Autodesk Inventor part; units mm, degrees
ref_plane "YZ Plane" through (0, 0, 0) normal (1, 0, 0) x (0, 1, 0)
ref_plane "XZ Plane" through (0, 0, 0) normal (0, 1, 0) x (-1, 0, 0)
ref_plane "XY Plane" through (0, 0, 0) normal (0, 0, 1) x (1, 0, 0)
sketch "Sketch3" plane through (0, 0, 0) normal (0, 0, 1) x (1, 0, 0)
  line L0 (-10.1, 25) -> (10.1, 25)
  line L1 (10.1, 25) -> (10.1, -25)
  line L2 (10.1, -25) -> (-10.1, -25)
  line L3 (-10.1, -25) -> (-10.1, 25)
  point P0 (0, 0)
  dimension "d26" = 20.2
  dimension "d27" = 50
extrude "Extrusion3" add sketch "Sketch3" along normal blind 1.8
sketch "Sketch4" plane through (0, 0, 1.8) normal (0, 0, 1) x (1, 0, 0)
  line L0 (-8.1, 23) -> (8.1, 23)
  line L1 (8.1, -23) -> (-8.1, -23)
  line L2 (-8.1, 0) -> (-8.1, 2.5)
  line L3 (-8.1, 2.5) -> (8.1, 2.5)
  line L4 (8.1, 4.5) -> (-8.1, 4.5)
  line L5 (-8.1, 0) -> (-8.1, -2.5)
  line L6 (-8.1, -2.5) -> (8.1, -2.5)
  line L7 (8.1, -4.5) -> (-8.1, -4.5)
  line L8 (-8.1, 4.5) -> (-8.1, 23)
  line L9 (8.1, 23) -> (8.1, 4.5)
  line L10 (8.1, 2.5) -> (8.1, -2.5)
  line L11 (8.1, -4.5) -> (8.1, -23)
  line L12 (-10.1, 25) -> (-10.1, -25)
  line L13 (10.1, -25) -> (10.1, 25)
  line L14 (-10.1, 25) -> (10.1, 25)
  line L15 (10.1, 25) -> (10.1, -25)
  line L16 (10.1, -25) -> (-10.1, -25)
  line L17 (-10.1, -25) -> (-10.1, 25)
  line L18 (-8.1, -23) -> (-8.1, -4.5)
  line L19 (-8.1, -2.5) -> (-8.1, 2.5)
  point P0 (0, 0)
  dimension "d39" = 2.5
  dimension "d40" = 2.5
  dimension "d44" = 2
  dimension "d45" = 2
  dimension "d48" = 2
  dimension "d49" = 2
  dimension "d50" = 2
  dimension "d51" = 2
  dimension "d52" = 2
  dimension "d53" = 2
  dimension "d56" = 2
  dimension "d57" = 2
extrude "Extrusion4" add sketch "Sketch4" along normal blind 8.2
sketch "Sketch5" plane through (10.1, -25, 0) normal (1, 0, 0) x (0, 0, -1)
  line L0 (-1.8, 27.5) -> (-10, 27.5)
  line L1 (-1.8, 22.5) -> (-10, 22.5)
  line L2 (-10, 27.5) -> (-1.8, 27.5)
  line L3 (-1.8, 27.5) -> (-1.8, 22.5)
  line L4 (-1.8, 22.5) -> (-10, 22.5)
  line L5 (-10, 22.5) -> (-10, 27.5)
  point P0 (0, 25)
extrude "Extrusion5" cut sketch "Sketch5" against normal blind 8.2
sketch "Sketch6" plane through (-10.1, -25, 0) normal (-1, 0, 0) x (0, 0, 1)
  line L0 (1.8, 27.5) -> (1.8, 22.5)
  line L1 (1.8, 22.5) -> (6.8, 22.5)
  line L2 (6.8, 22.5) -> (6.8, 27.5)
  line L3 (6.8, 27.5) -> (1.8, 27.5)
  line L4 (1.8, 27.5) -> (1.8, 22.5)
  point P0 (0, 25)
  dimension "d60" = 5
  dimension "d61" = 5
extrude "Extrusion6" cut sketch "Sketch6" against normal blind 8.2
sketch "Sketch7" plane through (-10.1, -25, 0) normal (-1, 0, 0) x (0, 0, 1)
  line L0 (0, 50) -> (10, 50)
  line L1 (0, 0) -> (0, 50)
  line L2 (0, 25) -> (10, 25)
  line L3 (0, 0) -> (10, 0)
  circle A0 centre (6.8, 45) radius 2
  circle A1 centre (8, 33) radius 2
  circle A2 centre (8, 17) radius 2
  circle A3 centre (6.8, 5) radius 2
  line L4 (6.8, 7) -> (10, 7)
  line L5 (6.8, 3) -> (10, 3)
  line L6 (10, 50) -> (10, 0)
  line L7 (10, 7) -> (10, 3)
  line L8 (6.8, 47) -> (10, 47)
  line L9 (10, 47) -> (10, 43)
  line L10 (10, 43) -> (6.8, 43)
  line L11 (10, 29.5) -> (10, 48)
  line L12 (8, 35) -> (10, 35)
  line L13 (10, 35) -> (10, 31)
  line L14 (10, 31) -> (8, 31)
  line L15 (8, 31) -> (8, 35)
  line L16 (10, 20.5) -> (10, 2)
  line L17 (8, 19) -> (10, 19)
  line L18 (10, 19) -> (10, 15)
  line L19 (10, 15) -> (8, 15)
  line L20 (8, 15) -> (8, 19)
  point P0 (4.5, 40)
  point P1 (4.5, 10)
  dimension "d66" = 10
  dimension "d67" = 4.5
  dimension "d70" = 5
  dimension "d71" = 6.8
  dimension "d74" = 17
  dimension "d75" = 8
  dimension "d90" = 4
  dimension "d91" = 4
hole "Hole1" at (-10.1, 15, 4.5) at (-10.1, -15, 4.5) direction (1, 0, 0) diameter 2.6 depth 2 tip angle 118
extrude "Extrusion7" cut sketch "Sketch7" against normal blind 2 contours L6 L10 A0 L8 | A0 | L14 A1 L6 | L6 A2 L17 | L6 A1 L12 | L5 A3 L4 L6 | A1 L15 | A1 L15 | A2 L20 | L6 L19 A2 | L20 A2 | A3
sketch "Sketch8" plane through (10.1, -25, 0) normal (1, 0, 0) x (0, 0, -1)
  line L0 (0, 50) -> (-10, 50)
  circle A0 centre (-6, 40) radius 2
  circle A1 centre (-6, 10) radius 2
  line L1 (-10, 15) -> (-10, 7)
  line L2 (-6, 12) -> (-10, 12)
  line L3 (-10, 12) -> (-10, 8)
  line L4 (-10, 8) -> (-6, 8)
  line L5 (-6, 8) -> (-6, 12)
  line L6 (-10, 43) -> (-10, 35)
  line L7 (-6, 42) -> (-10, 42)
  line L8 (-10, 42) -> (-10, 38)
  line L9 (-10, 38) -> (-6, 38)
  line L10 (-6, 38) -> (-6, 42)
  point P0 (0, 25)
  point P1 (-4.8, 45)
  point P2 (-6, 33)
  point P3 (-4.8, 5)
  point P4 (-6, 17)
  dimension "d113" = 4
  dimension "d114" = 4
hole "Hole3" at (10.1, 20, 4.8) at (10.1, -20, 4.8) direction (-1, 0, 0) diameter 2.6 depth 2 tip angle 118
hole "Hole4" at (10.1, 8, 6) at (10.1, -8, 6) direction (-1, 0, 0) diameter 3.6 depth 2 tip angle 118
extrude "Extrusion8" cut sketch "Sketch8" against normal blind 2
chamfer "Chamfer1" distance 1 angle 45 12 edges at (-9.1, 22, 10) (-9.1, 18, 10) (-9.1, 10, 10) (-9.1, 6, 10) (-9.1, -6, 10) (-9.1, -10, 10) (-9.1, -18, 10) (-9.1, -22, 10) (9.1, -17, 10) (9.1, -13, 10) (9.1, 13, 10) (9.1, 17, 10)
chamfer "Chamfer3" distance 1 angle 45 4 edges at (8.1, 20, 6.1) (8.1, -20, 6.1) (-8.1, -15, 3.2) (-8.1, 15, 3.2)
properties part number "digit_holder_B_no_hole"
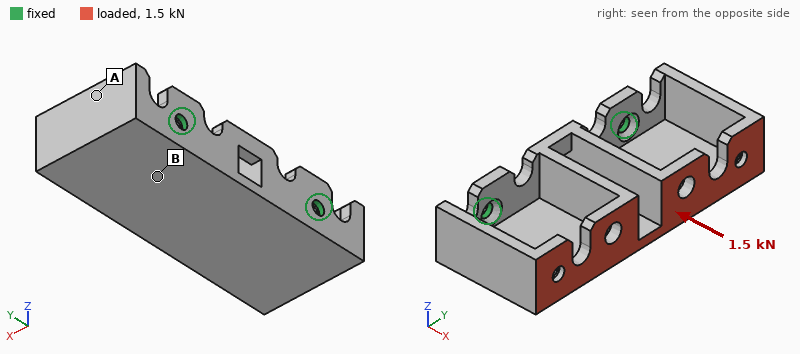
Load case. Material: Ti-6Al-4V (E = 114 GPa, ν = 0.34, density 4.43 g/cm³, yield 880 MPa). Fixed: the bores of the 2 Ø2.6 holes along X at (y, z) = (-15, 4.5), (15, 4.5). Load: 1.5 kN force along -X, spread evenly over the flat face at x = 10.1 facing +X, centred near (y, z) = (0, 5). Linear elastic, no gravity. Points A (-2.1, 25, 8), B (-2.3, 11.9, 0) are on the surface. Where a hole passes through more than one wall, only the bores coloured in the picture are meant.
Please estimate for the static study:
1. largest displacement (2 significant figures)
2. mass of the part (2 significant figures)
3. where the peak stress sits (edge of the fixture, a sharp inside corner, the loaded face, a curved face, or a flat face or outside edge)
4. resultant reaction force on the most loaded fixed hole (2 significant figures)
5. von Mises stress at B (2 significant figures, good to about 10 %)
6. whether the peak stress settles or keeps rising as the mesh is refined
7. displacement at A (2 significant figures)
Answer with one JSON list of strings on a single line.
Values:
["0.20 mm", "18 g", "edge of the fixture", "760 N", "41 MPa", "keeps rising", "0.078 mm"]
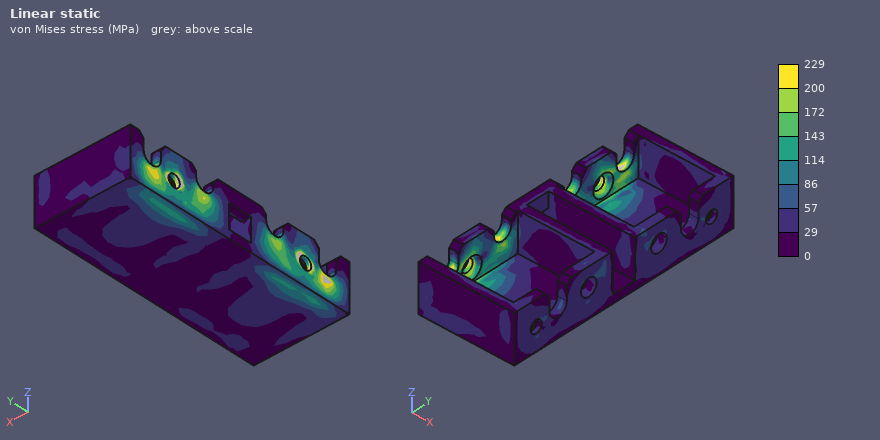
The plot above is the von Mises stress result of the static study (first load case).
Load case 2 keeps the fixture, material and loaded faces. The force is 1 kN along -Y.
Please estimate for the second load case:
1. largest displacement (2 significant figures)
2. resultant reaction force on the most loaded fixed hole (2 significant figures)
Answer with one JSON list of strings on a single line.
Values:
["0.16 mm", "820 N"]
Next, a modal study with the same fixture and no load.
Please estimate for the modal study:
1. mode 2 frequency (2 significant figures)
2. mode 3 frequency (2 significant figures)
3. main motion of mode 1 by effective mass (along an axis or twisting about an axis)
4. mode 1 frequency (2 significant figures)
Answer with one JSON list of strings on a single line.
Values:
["3500 Hz", "5900 Hz", "along Z", "1800 Hz"]
